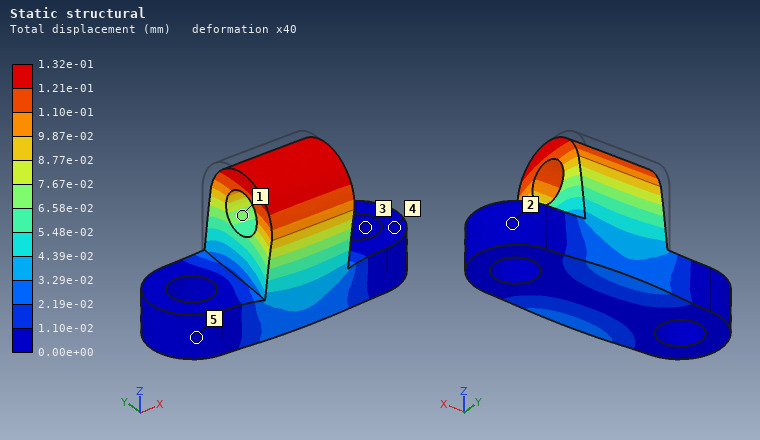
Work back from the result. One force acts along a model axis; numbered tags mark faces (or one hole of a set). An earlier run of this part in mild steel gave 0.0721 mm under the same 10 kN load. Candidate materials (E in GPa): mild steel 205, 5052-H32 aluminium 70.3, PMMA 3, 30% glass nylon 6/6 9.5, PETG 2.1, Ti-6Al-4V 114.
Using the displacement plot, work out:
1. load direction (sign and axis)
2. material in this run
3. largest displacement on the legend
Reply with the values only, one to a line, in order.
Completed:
-Y
Ti-6Al-4V
1.32e-01 mm
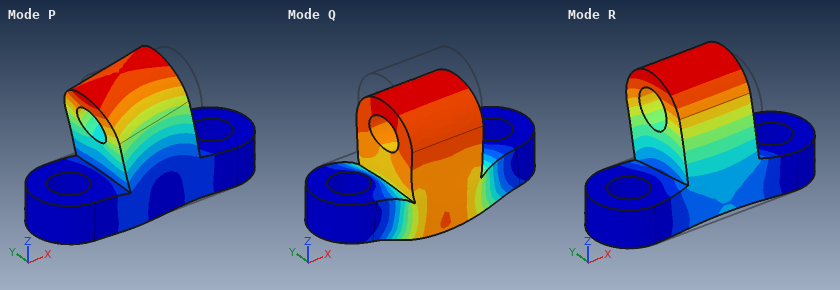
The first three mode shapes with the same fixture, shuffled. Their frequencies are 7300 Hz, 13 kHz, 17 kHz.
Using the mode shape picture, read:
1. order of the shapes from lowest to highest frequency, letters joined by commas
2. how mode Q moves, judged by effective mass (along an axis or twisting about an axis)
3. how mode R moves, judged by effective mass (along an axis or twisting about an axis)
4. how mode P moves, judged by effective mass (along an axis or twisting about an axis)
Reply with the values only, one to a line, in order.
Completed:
R, P, Q
along Z
along Y
along X
